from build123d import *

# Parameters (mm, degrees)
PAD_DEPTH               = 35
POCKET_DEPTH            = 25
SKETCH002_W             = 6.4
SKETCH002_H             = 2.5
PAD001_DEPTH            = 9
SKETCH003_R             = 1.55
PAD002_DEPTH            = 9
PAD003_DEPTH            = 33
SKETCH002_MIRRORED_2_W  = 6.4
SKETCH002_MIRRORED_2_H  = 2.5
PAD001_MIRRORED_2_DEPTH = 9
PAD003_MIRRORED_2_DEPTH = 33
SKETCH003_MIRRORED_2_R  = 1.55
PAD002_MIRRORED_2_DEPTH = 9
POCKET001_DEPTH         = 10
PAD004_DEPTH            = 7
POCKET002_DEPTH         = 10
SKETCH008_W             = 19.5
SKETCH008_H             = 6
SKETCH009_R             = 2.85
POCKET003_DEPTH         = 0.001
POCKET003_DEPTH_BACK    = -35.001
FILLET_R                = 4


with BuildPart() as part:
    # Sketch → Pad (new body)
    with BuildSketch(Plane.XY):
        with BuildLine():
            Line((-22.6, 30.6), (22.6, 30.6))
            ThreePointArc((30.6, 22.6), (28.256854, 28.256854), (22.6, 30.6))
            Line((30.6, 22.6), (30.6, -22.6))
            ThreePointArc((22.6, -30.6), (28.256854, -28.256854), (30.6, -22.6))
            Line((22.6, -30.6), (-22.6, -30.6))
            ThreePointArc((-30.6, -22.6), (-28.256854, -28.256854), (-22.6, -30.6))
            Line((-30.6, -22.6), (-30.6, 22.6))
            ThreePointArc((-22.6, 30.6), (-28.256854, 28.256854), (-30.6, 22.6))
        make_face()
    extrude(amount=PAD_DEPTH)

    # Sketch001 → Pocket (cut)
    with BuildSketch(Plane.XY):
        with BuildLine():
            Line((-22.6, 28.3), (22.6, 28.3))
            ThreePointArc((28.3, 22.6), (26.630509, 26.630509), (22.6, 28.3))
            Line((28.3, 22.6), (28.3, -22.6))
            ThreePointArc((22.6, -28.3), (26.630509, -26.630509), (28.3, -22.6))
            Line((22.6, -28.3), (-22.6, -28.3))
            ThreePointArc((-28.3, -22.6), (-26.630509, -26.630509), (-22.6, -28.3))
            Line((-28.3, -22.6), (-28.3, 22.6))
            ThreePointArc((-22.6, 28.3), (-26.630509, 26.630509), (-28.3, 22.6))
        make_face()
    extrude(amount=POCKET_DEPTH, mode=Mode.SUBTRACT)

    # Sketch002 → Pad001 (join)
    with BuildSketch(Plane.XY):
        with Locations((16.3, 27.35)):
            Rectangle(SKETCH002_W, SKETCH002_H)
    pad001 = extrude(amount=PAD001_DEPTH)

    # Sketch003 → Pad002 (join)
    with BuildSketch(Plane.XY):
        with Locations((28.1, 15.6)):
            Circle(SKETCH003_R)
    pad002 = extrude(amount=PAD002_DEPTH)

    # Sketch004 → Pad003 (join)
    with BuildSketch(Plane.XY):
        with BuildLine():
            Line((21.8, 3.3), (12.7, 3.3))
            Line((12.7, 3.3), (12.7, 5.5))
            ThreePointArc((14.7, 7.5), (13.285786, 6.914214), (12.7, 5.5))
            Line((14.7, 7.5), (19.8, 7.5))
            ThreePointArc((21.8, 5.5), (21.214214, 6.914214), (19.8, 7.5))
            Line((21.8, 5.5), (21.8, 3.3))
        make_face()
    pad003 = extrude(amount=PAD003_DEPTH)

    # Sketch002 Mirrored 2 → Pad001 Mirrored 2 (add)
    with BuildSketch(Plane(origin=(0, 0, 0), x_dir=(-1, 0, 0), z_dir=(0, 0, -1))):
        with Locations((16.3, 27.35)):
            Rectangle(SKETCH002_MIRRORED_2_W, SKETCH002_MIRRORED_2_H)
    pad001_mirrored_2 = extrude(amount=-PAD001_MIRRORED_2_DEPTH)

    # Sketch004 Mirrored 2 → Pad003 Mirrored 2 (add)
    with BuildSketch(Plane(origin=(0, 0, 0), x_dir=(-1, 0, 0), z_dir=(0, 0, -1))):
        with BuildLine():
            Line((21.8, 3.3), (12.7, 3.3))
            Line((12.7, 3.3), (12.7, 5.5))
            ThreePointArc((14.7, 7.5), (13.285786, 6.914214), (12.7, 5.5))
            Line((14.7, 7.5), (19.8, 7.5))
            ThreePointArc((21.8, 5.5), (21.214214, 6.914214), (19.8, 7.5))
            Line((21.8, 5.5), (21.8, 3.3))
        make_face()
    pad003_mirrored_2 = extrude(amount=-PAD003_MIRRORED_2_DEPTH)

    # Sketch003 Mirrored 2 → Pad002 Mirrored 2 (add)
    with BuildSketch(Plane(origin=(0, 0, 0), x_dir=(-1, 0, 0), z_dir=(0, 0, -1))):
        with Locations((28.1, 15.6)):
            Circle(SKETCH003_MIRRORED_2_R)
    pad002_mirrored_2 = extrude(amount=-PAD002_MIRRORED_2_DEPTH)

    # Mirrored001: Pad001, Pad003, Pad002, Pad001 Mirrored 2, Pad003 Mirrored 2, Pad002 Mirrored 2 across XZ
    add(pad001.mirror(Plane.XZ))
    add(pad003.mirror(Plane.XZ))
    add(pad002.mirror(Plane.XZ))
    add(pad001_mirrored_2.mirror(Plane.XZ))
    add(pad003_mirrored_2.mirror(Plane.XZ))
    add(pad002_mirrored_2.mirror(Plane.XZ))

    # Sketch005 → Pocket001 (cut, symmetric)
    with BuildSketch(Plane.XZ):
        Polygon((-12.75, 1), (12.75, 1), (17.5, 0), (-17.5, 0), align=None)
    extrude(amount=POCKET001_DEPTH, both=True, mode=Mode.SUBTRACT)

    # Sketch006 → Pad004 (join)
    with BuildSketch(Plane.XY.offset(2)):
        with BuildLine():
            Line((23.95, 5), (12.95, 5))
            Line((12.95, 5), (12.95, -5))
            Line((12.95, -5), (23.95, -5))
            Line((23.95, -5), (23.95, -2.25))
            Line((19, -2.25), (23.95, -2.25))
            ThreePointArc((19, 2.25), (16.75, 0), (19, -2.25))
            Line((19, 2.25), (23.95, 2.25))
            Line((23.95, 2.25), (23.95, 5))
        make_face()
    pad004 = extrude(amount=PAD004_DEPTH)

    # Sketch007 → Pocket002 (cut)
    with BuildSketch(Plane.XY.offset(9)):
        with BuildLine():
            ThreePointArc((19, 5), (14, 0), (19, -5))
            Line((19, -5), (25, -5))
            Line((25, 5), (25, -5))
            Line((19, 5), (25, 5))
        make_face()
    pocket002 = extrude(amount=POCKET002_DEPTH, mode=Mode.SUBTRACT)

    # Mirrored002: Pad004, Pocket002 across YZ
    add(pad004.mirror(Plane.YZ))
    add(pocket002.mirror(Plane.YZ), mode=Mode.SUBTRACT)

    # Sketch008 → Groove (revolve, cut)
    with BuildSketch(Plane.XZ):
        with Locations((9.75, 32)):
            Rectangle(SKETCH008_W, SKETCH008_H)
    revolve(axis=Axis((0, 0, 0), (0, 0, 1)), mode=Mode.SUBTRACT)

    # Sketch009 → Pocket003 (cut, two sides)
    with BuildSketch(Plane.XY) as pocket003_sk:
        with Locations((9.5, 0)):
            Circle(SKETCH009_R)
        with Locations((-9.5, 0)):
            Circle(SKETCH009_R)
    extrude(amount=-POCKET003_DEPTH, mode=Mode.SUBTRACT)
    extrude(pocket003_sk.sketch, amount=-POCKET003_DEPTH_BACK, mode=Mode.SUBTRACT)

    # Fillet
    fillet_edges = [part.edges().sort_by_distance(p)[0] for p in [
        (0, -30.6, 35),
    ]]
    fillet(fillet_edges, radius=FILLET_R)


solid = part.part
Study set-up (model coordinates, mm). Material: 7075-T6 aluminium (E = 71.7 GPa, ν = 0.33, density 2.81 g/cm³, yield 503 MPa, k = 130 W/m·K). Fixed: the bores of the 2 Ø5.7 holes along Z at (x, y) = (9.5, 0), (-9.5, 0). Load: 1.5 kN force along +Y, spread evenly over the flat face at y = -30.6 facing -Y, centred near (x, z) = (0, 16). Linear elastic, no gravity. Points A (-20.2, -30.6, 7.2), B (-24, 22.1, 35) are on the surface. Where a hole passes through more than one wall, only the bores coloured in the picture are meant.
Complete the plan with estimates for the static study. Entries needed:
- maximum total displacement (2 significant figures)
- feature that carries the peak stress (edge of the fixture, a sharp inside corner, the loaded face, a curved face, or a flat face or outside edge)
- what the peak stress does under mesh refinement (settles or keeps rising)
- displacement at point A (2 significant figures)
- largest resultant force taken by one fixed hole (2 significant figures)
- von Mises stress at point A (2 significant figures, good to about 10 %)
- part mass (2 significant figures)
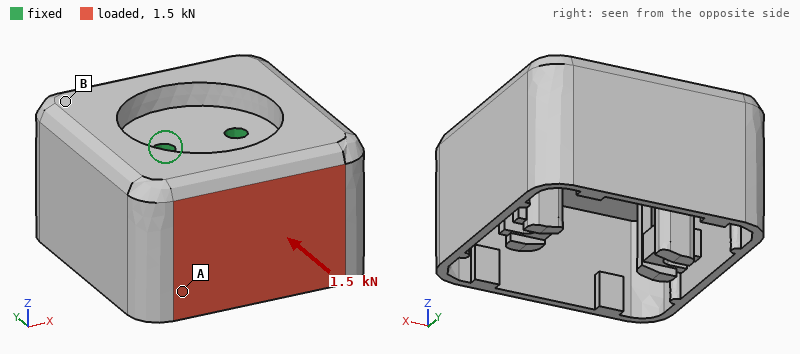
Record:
0.37 mm
edge of the fixture
keeps rising
0.16 mm
780 N
63 MPa
130 g
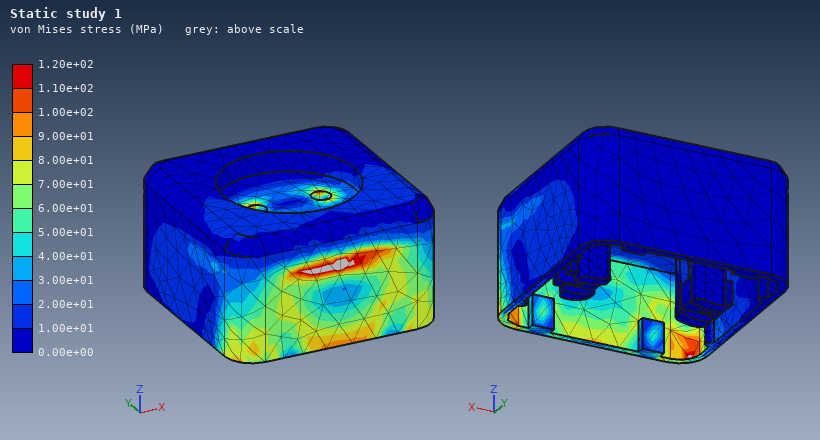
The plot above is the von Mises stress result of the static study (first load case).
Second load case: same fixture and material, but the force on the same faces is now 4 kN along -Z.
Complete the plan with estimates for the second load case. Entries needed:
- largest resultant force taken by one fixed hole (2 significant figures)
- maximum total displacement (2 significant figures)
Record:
2.0 kN
0.85 mm
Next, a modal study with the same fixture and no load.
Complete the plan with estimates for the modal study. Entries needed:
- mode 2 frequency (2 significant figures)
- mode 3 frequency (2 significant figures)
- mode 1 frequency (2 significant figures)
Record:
2800 Hz
3600 Hz
1700 Hz
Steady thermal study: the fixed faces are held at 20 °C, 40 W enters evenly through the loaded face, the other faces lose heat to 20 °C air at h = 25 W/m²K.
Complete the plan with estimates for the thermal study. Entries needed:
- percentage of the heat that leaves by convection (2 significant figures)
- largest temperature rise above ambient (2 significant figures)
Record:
17 %
43 K
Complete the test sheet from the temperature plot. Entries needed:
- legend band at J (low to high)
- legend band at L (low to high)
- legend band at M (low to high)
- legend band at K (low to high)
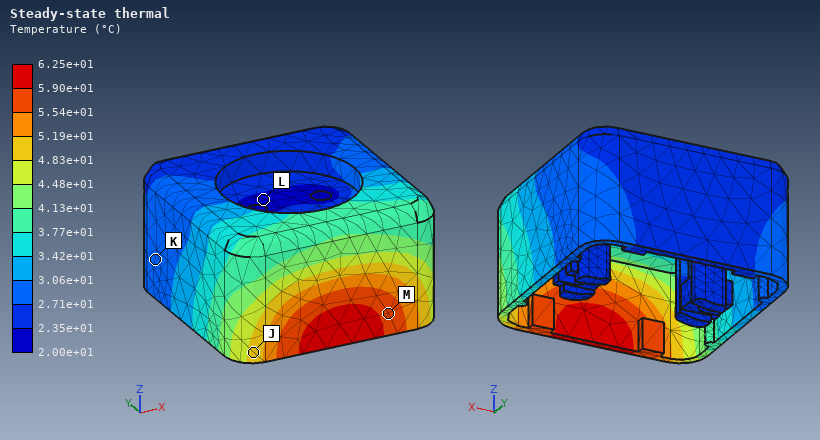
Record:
4.83e+01 to 5.19e+01 °C
2.00e+01 to 2.35e+01 °C
5.54e+01 to 5.90e+01 °C
2.71e+01 to 3.06e+01 °C
